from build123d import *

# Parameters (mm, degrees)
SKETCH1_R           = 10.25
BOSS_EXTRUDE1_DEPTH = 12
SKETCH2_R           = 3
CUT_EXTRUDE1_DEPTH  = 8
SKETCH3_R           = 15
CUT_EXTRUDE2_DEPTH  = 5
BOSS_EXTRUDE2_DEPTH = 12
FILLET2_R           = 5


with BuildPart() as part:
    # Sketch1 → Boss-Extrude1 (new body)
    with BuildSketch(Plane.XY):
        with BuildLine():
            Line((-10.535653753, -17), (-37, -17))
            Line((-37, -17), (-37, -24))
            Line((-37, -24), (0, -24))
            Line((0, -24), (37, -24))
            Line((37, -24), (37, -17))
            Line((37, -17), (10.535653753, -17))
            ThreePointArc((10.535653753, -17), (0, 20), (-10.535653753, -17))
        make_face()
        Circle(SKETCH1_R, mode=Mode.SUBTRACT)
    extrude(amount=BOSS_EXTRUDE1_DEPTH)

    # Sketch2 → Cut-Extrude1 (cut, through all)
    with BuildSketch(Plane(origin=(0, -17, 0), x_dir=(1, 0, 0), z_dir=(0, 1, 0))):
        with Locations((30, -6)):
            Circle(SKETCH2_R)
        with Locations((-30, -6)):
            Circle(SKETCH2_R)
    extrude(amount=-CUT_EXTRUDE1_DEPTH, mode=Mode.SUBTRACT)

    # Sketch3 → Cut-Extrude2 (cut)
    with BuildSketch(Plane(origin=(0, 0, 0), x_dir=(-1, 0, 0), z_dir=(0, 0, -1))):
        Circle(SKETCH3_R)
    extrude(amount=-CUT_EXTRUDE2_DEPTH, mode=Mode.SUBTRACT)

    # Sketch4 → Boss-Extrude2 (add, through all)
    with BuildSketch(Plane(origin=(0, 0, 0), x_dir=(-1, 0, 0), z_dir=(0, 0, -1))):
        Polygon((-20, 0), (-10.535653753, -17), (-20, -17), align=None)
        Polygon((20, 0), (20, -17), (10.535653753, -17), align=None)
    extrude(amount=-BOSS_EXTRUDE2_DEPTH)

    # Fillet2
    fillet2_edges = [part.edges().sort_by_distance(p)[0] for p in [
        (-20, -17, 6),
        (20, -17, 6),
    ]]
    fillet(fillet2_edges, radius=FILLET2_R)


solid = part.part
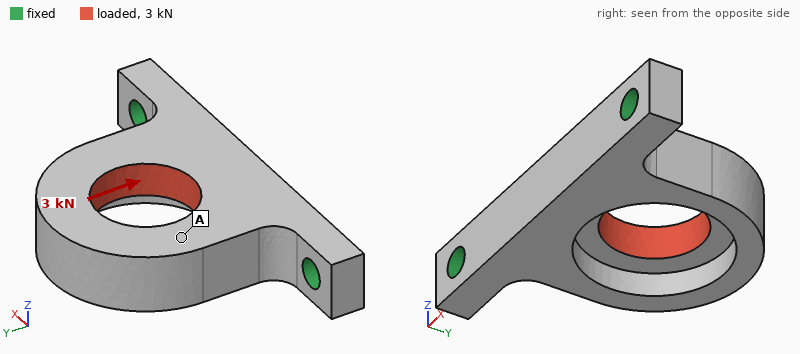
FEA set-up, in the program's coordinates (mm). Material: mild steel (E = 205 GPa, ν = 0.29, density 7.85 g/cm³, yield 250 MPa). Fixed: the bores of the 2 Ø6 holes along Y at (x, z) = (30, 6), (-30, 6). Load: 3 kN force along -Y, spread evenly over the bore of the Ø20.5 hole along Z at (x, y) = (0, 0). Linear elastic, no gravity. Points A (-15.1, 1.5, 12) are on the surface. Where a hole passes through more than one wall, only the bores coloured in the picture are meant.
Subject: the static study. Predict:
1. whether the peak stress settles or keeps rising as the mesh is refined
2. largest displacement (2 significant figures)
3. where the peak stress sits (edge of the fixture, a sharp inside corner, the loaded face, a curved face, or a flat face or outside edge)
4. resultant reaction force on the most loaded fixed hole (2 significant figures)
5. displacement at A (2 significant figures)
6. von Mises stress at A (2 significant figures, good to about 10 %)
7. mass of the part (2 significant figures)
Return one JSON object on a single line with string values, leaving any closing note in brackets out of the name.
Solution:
{"whether the peak stress settles or keeps rising as the mesh is refined": "keeps rising", "largest displacement": "25 µm", "where the peak stress sits": "edge of the fixture", "resultant reaction force on the most loaded fixed hole": "1.7 kN", "displacement at A": "14 µm", "von Mises stress at A": "17 MPa", "mass of the part": "120 g"}
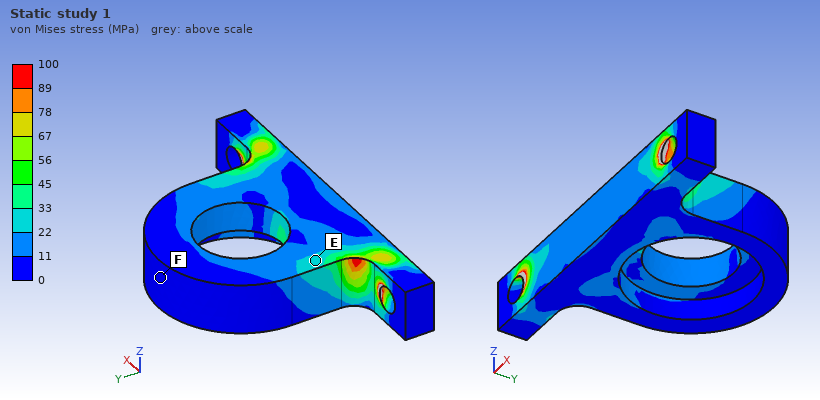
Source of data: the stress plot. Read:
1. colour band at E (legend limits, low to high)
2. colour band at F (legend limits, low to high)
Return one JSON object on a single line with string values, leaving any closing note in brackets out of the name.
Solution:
{"colour band at E": "22 to 33 MPa", "colour band at F": "0 to 11 MPa"}
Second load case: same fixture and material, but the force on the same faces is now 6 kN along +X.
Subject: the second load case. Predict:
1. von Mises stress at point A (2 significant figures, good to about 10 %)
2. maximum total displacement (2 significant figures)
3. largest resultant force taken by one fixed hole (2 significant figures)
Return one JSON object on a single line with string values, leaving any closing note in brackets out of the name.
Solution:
{"von Mises stress at point A": "42 MPa", "maximum total displacement": "28 µm", "largest resultant force taken by one fixed hole": "3.9 kN"}
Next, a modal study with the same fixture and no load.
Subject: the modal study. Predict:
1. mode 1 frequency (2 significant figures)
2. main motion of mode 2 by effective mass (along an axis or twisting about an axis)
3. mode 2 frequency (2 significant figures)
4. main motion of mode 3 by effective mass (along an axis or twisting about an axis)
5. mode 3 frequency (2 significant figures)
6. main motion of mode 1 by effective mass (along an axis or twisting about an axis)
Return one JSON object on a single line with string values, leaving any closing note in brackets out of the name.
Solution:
{"mode 1 frequency": "2900 Hz", "main motion of mode 2 by effective mass": "along X", "mode 2 frequency": "8800 Hz", "main motion of mode 3 by effective mass": "along X", "mode 3 frequency": "10 kHz", "main motion of mode 1 by effective mass": "along Z"}
